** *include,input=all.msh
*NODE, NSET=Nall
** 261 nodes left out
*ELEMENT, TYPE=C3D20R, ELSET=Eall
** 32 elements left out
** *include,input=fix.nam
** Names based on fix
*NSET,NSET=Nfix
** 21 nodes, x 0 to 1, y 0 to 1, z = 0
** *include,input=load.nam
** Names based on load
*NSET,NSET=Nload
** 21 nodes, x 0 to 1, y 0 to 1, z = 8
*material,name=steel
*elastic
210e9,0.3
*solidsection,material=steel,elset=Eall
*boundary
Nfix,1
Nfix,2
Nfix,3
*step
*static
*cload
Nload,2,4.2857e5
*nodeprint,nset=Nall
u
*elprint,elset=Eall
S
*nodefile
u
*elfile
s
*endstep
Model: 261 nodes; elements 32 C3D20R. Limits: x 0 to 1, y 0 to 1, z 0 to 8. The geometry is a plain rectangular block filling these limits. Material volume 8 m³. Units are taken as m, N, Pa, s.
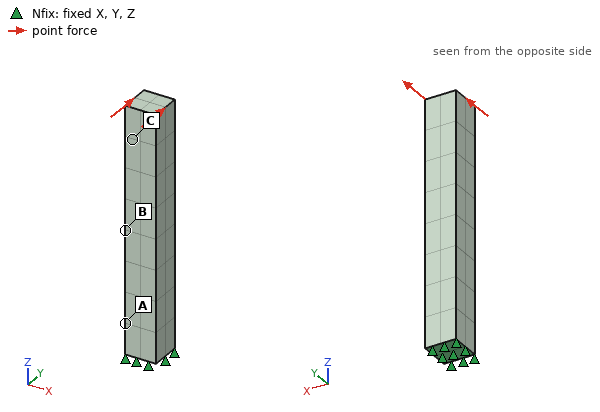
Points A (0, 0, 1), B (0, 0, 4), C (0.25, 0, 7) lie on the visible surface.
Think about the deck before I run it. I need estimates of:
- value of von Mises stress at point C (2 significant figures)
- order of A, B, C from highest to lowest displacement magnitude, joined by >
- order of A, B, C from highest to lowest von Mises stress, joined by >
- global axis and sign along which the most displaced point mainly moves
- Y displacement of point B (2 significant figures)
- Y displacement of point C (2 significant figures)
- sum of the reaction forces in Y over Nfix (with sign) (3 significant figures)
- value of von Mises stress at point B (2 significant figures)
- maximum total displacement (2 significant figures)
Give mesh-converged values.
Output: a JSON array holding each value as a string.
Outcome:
["5.3e+07 Pa", "C > B > A", "A > B > C", "+Y", "0.028 m", "0.072 m", "-9.00e+06 N", "2.2e+08 Pa", "0.088 m"]
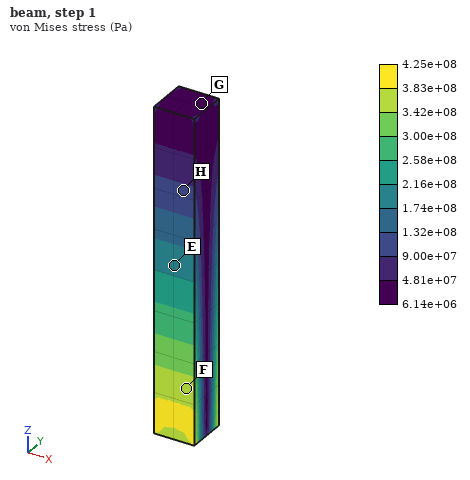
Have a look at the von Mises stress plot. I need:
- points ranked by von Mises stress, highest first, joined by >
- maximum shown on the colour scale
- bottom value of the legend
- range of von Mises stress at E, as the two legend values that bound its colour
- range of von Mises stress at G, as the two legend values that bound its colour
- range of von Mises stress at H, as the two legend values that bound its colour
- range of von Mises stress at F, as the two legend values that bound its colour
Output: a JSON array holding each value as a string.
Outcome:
["F > E > H > G", "4.25e+08 Pa", "6.14e+06 Pa", "1.74e+08 to 2.16e+08 Pa", "6.14e+06 to 4.81e+07 Pa", "9.00e+07 to 1.32e+08 Pa", "3.42e+08 to 3.83e+08 Pa"]
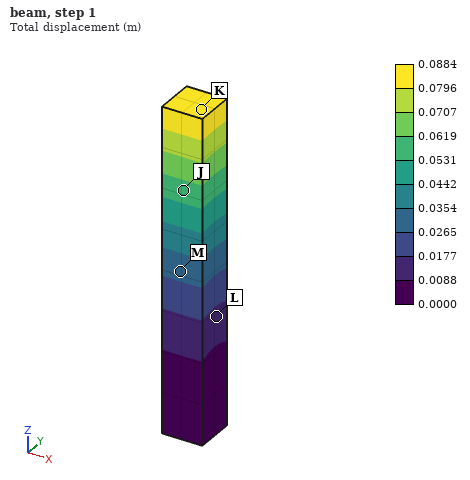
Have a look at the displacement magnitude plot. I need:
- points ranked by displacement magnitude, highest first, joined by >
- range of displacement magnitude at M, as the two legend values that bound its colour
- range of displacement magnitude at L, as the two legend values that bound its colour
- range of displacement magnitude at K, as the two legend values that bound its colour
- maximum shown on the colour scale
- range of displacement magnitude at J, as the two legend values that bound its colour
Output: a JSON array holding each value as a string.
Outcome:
["K > J > M > L", "0.0265 to 0.0354 m", "0.0088 to 0.0177 m", "0.0796 to 0.0884 m", "0.0884 m", "0.0531 to 0.0619 m"]
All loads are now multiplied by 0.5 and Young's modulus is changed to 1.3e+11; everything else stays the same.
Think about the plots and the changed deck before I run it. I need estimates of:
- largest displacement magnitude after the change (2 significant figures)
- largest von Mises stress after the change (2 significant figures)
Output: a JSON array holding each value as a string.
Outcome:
["0.071 m", "2.1e+08 Pa"]
